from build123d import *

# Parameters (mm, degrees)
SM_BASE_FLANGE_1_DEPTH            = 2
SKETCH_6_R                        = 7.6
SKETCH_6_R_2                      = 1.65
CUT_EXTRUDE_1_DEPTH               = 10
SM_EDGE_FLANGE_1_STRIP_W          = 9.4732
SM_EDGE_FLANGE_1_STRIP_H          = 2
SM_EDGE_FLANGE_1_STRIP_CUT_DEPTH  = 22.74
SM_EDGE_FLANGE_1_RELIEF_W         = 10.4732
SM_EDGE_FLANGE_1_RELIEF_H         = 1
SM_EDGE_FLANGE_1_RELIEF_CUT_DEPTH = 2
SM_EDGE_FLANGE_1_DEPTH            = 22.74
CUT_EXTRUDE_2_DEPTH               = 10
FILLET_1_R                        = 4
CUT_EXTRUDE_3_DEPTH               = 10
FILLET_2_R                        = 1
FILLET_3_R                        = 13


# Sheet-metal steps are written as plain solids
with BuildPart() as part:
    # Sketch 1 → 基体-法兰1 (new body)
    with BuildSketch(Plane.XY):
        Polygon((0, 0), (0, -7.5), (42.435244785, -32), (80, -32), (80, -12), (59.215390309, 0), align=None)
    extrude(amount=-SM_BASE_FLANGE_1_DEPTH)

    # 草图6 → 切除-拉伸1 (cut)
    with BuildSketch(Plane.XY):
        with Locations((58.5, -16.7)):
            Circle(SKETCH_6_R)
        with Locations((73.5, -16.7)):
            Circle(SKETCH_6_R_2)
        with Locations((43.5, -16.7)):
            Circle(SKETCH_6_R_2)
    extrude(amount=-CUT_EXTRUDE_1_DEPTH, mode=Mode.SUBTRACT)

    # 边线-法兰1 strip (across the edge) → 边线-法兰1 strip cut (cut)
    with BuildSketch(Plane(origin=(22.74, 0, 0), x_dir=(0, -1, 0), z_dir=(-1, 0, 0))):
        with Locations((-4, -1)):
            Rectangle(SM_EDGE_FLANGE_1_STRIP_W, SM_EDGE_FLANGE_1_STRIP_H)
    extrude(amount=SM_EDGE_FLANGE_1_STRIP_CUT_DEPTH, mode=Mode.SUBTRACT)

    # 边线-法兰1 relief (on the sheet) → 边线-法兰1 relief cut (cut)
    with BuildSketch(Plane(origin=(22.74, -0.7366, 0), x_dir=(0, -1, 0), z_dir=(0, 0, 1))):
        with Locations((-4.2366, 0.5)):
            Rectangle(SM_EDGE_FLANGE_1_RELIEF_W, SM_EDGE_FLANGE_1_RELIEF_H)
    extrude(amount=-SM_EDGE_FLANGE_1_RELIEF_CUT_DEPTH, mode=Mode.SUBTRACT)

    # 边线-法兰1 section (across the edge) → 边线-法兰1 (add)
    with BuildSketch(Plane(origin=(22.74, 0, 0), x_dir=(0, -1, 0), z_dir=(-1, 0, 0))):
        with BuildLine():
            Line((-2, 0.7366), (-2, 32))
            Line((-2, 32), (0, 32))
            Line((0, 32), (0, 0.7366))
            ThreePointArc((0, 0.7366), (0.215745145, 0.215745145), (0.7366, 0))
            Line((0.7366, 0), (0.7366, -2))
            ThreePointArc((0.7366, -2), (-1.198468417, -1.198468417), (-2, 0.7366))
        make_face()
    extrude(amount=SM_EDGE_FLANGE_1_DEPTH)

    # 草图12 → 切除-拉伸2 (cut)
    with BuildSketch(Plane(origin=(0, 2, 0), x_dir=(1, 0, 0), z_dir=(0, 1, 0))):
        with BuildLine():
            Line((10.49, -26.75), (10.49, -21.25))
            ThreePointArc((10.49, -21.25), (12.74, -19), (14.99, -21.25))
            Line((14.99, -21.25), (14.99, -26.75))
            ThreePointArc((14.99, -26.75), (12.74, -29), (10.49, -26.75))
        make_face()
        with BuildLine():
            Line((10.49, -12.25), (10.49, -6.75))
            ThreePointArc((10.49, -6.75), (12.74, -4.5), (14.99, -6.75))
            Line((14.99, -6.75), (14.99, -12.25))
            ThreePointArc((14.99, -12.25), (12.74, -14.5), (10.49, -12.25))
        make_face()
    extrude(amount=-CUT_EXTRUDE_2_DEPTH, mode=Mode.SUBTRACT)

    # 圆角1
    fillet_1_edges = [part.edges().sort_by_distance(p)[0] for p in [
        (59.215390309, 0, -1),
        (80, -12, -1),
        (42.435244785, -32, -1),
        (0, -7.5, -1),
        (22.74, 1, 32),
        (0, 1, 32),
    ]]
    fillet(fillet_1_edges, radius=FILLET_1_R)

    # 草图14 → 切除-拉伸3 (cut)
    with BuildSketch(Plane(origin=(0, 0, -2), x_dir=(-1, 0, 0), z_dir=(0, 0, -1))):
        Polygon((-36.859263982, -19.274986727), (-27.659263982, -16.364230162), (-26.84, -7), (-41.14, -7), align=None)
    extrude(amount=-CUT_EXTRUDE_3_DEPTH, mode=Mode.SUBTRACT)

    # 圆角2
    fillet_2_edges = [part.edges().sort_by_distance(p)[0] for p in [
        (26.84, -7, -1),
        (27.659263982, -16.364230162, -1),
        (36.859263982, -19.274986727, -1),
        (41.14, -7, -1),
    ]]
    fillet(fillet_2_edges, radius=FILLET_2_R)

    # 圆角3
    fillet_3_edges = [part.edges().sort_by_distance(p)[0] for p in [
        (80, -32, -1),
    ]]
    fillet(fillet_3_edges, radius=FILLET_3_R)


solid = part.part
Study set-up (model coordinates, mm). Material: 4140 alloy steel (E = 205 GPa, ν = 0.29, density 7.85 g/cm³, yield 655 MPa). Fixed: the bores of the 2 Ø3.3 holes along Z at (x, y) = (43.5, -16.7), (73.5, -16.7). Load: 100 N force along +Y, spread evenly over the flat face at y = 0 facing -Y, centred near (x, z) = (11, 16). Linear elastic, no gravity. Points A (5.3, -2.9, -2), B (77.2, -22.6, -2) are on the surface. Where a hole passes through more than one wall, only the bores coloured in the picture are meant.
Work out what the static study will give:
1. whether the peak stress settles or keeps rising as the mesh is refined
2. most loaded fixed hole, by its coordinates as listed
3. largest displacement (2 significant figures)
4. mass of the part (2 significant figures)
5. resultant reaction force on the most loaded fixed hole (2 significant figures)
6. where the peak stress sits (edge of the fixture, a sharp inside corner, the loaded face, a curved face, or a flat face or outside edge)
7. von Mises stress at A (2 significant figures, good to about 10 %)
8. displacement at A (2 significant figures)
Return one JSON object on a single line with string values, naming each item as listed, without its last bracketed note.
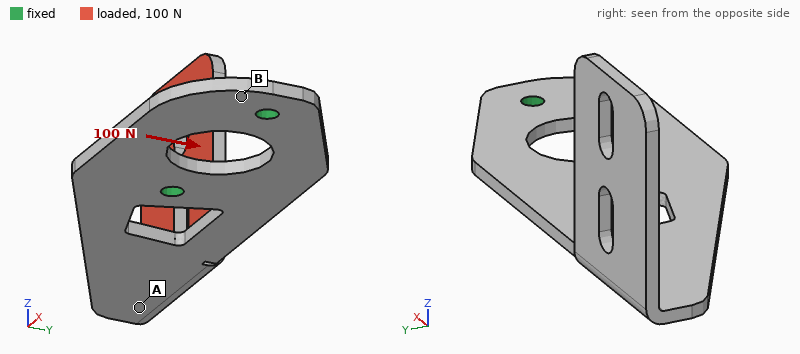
{"whether the peak stress settles or keeps rising as the mesh is refined": "keeps rising", "most loaded fixed hole, by its coordinates as listed": "(43.5, -16.7)", "largest displacement": "0.88 mm", "mass of the part": "35 g", "resultant reaction force on the most loaded fixed hole": "190 N", "where the peak stress sits": "a sharp inside corner", "von Mises stress at A": "78 MPa", "displacement at A": "0.22 mm"}
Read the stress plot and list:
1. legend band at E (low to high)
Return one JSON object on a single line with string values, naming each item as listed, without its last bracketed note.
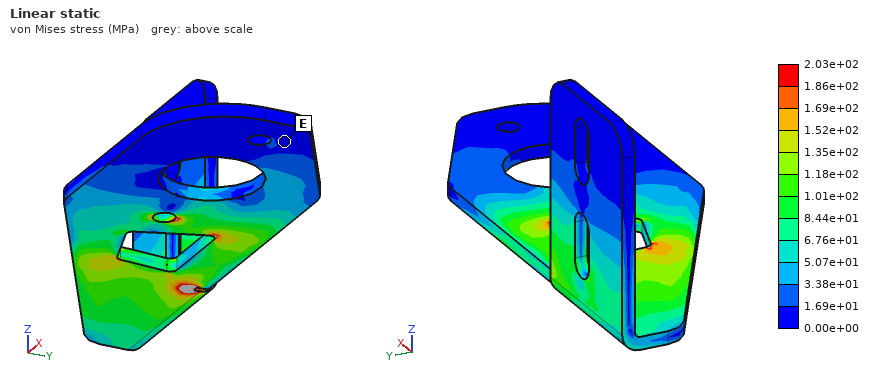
{"legend band at E": "0.00e+00 to 1.69e+01 MPa"}
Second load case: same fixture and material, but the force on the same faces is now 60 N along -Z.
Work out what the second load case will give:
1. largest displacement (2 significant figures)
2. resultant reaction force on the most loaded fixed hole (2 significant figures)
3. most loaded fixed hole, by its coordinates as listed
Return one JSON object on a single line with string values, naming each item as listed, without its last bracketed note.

{"largest displacement": "0.90 mm", "resultant reaction force on the most loaded fixed hole": "86 N", "most loaded fixed hole, by its coordinates as listed": "(43.5, -16.7)"}
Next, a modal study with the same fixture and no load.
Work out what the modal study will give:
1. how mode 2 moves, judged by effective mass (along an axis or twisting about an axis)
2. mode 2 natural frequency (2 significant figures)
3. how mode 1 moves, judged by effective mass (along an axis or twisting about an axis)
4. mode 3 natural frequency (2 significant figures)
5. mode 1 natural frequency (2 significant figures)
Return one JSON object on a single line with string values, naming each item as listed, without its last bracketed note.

{"how mode 2 moves, judged by effective mass": "along Y", "mode 2 natural frequency": "730 Hz", "how mode 1 moves, judged by effective mass": "along Z", "mode 3 natural frequency": "1600 Hz", "mode 1 natural frequency": "380 Hz"}
